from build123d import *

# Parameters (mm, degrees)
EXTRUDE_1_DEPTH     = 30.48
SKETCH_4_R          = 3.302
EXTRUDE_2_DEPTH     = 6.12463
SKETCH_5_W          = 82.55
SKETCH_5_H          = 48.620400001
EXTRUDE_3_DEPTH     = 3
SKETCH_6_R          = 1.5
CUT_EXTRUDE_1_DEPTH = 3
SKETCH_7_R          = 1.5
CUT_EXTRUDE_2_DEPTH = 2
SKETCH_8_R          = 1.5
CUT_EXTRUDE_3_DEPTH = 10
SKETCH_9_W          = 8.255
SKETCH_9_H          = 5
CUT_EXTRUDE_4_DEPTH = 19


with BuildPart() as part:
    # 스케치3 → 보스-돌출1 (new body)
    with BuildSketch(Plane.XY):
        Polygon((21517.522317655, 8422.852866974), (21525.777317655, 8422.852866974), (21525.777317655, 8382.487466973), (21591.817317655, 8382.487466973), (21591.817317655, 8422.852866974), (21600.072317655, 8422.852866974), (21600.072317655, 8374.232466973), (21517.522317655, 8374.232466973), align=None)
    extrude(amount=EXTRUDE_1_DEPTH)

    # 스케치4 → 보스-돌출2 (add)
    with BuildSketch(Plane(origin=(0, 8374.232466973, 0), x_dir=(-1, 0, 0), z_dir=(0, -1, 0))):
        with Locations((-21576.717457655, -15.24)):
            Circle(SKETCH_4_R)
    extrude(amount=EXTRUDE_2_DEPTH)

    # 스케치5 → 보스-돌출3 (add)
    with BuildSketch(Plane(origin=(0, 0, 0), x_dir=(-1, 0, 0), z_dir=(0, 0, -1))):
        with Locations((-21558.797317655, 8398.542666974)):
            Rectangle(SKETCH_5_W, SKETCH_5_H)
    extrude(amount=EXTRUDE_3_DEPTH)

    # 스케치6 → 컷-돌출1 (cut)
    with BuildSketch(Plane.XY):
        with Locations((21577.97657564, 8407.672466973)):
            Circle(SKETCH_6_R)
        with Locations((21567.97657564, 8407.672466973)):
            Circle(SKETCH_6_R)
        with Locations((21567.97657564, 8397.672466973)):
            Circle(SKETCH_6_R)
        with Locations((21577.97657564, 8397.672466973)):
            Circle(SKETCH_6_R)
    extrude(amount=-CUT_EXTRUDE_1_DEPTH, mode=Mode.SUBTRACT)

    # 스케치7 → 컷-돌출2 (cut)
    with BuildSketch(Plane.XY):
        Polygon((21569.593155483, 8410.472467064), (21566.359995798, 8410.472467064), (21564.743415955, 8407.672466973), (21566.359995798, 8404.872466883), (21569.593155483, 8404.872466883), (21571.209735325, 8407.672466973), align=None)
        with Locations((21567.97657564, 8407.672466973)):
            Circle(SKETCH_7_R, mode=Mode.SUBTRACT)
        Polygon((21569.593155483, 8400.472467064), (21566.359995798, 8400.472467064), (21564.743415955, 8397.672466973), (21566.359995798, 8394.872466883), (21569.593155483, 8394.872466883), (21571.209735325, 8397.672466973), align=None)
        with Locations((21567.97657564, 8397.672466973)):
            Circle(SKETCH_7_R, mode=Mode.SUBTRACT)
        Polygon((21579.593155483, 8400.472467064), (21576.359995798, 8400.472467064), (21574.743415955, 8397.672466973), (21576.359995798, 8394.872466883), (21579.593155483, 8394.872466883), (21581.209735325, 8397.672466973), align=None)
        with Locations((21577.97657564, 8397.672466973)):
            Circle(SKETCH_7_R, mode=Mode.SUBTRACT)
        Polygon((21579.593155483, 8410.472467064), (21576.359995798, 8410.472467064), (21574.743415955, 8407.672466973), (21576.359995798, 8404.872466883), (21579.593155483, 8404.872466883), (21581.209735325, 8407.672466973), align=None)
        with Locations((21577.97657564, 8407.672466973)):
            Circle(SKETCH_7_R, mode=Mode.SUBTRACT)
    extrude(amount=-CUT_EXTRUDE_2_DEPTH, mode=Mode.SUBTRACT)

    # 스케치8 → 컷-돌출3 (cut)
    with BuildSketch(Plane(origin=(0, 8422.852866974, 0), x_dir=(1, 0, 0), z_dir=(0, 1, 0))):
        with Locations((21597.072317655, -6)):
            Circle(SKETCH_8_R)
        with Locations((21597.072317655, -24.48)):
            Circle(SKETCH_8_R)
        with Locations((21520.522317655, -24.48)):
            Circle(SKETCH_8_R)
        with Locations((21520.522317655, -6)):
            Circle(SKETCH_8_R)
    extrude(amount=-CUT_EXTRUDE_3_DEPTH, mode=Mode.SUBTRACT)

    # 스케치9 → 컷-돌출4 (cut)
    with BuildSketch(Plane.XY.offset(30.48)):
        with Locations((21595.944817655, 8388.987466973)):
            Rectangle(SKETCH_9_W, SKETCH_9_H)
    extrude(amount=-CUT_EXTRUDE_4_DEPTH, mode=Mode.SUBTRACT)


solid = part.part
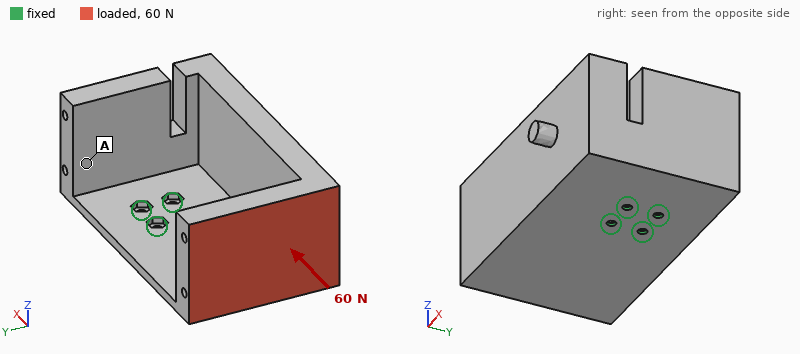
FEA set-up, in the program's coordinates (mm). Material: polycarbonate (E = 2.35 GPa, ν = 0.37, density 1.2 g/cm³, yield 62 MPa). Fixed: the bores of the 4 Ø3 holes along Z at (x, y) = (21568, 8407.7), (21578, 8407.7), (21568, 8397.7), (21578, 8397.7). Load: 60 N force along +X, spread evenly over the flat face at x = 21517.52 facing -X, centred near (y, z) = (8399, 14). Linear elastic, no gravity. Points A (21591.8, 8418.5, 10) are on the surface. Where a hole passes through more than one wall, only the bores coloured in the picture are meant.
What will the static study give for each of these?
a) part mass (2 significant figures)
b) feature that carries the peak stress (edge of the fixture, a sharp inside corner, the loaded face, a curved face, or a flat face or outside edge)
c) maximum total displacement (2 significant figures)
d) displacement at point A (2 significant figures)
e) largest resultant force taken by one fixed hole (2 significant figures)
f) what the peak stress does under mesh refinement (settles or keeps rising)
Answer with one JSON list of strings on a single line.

["62 g", "edge of the fixture", "1.2 mm", "0.28 mm", "64 N", "keeps rising"]
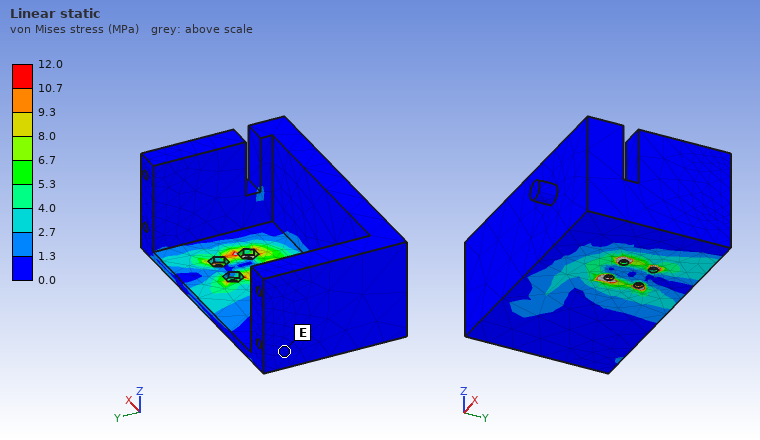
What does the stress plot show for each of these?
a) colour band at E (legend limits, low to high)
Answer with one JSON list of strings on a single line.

["0.0 to 1.3 MPa"]
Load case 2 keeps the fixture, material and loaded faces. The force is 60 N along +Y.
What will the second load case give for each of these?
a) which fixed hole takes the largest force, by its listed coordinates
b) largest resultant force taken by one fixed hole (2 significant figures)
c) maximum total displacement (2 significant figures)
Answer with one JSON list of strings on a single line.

["(21568, 8407.7)", "150 N", "1.2 mm"]
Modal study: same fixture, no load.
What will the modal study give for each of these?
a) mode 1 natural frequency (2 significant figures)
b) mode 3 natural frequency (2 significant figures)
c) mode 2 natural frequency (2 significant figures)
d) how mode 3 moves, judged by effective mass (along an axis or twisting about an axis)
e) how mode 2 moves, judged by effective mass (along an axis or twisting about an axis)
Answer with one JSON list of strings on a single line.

["130 Hz", "470 Hz", "190 Hz", "along Z", "along Y"]
